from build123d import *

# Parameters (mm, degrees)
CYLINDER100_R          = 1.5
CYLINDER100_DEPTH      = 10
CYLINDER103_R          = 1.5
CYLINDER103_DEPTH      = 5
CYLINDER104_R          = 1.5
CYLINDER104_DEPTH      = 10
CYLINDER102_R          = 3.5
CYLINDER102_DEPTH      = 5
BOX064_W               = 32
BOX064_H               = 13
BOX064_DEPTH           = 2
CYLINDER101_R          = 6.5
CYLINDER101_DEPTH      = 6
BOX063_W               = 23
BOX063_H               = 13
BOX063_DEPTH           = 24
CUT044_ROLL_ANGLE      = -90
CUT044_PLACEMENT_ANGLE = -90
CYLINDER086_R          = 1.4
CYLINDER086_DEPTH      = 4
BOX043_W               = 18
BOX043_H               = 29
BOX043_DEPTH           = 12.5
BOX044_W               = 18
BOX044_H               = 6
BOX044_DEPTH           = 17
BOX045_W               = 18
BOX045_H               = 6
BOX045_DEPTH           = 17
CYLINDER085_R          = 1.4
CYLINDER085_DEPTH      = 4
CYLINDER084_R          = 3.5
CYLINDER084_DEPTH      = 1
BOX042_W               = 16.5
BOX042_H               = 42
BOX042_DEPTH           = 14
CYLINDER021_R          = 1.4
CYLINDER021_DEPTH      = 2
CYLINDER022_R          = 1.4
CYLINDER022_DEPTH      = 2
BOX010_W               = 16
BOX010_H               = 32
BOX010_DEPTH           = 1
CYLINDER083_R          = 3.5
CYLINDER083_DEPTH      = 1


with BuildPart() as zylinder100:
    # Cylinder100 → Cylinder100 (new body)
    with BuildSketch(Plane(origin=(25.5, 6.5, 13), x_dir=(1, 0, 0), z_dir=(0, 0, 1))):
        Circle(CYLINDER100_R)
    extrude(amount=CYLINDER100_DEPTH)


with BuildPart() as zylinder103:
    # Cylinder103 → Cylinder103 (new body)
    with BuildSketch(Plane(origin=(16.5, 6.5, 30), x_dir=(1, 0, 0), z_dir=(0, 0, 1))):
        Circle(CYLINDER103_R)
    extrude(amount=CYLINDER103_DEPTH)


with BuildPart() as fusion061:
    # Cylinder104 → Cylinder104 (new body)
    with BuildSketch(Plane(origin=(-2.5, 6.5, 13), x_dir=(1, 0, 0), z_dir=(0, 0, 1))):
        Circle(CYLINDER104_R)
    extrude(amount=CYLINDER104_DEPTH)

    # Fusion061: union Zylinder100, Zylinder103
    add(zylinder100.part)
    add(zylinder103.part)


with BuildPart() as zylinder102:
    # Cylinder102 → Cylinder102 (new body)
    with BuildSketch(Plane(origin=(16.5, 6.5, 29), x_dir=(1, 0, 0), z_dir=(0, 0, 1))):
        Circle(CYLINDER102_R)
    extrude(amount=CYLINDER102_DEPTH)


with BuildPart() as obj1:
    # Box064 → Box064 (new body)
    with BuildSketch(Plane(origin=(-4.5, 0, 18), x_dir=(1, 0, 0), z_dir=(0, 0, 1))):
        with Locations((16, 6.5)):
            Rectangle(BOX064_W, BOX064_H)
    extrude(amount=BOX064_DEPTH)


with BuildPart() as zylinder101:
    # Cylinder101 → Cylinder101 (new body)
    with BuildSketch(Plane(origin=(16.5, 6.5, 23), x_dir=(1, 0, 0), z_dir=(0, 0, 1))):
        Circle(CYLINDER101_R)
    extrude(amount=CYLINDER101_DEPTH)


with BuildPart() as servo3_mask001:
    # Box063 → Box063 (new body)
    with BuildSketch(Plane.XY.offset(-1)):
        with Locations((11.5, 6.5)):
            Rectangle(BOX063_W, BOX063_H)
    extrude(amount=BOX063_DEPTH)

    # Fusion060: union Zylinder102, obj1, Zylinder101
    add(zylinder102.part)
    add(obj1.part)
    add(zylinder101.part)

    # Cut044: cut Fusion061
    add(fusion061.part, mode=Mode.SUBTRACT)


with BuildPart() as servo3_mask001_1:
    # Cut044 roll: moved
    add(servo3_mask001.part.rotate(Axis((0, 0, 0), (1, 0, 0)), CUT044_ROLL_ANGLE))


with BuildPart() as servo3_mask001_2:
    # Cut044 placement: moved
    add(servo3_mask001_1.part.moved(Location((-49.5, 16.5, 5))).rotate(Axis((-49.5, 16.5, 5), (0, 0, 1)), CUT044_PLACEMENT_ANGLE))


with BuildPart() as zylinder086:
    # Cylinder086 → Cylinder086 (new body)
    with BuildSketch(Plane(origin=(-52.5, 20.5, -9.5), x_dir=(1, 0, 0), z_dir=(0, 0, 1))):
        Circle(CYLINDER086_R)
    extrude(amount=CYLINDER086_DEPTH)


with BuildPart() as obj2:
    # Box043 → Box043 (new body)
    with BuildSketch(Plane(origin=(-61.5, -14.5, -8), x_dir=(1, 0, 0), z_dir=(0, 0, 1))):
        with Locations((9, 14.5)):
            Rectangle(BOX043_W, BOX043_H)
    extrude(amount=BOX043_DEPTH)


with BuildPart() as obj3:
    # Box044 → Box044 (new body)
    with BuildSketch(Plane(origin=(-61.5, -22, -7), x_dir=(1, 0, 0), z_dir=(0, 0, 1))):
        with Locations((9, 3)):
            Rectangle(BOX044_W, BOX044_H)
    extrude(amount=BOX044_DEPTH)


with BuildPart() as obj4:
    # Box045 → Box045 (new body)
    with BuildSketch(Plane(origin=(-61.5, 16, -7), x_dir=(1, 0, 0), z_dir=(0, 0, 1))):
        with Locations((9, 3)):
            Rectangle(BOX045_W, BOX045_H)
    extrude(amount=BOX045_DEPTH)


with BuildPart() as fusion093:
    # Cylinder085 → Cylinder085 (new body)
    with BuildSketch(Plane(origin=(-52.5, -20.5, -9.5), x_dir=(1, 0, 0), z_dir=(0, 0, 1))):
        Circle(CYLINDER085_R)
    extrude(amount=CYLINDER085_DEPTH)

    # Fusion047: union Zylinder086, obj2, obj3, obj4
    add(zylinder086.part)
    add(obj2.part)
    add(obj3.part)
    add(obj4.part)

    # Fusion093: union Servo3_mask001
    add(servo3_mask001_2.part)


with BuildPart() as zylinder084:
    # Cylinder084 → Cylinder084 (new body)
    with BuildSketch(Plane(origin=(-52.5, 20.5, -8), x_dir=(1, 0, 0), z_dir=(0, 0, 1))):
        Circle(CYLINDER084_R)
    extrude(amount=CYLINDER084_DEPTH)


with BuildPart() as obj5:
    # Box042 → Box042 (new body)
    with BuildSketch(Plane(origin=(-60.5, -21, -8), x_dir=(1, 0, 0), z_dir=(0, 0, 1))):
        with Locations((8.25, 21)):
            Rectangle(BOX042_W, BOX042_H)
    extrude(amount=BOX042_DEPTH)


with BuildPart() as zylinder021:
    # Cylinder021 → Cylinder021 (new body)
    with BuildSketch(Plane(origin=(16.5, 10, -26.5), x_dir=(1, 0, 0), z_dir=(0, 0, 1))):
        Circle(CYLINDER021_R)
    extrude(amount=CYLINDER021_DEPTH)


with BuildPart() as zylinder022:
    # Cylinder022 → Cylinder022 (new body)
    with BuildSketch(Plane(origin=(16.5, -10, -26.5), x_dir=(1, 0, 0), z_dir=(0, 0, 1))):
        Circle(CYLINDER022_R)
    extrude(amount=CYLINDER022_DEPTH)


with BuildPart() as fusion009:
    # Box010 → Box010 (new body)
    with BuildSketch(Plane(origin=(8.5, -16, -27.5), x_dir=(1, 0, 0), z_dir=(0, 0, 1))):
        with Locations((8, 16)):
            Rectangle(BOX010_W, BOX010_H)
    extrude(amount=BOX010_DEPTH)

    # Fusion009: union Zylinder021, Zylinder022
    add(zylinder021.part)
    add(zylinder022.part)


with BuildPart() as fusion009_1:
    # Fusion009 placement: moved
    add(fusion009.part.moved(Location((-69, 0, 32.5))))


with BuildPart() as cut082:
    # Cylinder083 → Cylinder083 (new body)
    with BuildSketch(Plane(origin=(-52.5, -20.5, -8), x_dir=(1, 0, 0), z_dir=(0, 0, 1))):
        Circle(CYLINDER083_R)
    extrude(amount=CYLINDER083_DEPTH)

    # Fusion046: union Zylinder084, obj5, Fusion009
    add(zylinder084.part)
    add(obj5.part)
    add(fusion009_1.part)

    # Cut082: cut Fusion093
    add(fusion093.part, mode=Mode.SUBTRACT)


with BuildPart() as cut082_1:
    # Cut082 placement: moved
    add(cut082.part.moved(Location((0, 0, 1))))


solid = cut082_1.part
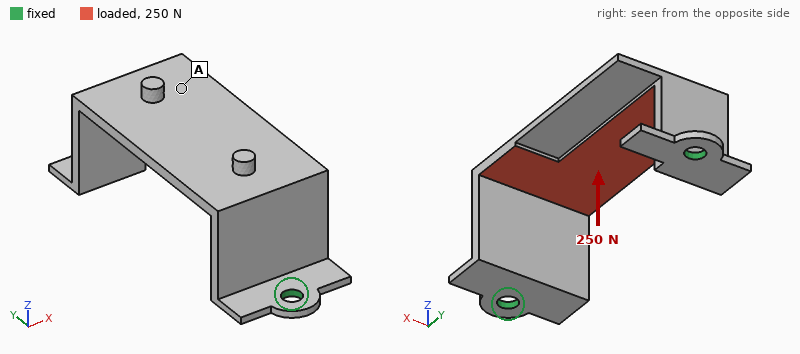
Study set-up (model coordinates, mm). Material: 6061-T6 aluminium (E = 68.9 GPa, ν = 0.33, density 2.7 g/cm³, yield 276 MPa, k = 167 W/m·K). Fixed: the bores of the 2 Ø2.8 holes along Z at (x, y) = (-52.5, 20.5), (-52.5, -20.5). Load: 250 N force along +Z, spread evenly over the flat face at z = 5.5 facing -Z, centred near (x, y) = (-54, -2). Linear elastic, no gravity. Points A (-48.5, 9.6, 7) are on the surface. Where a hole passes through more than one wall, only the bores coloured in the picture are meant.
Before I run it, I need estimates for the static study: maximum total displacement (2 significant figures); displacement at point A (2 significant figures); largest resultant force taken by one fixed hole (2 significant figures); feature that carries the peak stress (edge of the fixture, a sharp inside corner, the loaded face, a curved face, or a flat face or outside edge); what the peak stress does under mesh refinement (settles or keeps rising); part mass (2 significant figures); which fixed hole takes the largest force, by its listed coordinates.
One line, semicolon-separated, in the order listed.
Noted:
0.20 mm; 0.099 mm; 150 N; edge of the fixture; keeps rising; 3.8 g; (-52.5, -20.5)
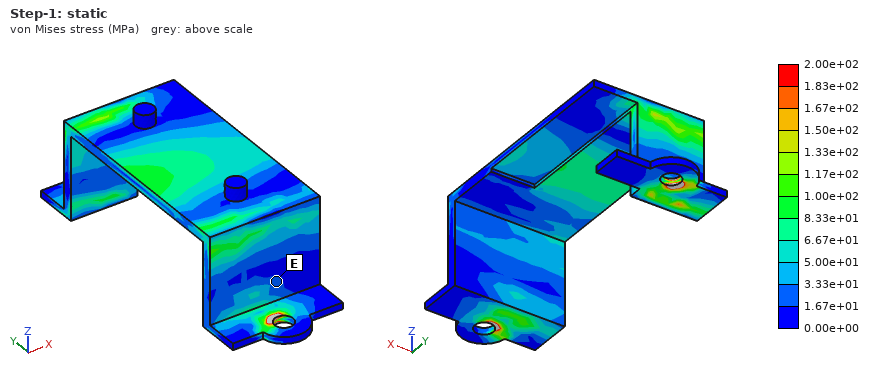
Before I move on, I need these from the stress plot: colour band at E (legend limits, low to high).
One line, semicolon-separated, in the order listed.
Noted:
1.67e+01 to 3.33e+01 MPa
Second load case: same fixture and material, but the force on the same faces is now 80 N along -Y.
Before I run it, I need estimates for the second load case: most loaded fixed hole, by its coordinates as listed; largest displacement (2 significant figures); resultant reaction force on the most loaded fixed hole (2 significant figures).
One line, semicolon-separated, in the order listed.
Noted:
(-52.5, -20.5); 0.11 mm; 48 N
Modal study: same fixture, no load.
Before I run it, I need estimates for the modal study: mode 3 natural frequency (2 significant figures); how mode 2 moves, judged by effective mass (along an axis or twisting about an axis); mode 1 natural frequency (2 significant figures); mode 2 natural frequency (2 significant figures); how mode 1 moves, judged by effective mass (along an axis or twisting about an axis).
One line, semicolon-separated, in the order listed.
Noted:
3900 Hz; along Y; 1900 Hz; 2800 Hz; along X
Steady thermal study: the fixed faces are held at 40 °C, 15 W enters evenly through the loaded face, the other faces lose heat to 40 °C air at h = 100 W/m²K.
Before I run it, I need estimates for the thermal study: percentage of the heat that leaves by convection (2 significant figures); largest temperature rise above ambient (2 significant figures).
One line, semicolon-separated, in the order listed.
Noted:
36 %; 47 K
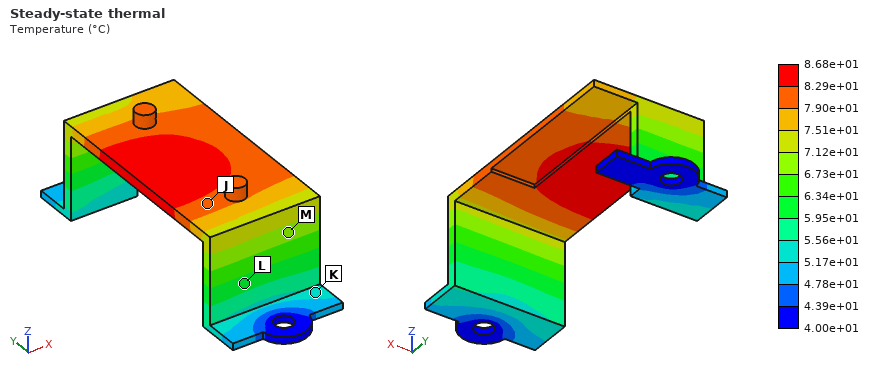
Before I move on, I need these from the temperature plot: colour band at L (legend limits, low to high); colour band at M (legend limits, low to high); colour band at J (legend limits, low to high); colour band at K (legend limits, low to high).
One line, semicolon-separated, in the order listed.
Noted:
5.95e+01 to 6.34e+01 °C; 6.73e+01 to 7.12e+01 °C; 7.90e+01 to 8.29e+01 °C; 5.17e+01 to 5.56e+01 °C
